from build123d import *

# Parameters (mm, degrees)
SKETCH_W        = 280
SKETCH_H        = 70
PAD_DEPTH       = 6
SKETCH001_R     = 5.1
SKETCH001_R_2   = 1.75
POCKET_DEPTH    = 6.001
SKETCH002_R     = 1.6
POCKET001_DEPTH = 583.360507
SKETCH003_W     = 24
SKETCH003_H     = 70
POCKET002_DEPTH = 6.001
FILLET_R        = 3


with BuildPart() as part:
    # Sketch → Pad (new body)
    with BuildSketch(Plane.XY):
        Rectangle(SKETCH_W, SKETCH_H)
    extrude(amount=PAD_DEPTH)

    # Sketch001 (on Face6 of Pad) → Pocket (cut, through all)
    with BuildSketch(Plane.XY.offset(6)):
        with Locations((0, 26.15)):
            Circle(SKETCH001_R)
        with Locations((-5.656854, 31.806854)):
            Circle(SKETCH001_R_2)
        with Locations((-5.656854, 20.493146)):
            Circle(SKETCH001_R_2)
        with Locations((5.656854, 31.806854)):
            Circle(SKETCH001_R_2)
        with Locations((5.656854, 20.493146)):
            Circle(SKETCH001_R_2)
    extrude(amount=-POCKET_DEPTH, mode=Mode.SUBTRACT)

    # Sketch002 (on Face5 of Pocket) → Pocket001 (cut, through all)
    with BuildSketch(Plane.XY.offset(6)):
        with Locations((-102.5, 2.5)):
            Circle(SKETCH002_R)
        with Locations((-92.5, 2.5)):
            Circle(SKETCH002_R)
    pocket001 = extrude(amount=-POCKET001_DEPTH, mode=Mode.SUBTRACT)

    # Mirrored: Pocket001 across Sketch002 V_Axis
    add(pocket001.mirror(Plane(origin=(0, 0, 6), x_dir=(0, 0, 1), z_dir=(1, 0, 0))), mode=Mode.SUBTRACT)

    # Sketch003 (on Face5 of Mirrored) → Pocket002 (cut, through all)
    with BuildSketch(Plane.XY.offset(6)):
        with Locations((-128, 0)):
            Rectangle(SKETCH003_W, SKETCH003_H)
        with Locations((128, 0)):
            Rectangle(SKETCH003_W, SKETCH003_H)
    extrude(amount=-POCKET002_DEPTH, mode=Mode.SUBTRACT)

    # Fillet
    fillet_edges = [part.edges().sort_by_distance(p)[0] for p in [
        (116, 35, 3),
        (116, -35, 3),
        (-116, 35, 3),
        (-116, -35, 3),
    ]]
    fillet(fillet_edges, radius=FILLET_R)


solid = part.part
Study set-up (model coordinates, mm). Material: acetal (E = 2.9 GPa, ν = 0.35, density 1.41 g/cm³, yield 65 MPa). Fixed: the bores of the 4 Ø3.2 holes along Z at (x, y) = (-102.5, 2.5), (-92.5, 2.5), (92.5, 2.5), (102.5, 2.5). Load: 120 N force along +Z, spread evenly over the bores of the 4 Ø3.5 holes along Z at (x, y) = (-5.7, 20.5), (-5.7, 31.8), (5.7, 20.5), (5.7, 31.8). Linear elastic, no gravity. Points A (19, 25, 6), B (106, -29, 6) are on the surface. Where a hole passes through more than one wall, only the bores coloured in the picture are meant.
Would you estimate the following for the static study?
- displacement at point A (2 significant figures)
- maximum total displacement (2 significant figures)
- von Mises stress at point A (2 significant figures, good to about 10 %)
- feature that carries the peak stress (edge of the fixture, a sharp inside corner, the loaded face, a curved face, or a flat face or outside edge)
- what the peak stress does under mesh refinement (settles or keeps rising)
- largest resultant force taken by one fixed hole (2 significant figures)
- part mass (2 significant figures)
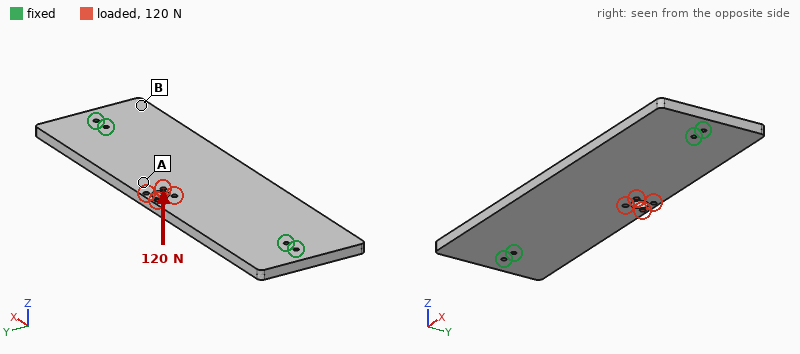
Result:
1.9 mm
2.5 mm
6.0 MPa
edge of the fixture
keeps rising
180 N
140 g
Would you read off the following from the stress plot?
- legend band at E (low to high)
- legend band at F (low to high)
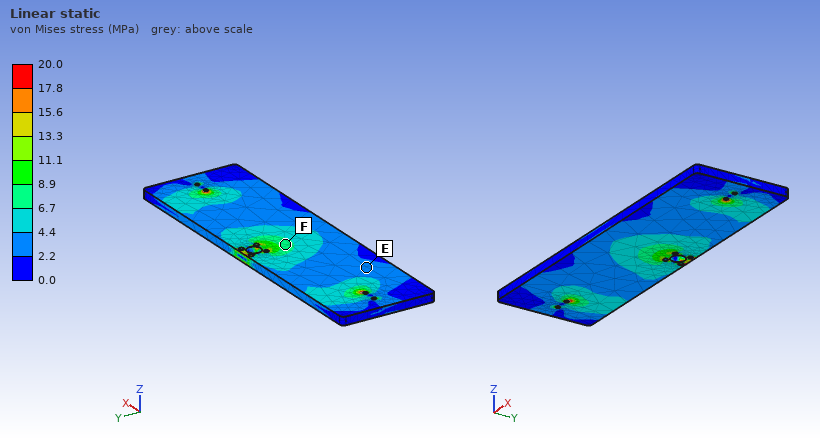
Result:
2.2 to 4.4 MPa
6.7 to 8.9 MPa
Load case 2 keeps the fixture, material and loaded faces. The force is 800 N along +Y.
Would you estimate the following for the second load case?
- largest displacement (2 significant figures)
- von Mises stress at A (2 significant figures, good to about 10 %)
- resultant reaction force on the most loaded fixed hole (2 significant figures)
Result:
0.35 mm
3.2 MPa
680 N
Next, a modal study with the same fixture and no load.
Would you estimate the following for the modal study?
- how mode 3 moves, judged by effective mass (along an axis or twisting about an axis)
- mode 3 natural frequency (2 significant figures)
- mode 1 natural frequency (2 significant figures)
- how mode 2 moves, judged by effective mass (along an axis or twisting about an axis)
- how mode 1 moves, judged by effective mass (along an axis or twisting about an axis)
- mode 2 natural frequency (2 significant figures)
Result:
twisting about Y
600 Hz
230 Hz
twisting about X
along Z
360 Hz
